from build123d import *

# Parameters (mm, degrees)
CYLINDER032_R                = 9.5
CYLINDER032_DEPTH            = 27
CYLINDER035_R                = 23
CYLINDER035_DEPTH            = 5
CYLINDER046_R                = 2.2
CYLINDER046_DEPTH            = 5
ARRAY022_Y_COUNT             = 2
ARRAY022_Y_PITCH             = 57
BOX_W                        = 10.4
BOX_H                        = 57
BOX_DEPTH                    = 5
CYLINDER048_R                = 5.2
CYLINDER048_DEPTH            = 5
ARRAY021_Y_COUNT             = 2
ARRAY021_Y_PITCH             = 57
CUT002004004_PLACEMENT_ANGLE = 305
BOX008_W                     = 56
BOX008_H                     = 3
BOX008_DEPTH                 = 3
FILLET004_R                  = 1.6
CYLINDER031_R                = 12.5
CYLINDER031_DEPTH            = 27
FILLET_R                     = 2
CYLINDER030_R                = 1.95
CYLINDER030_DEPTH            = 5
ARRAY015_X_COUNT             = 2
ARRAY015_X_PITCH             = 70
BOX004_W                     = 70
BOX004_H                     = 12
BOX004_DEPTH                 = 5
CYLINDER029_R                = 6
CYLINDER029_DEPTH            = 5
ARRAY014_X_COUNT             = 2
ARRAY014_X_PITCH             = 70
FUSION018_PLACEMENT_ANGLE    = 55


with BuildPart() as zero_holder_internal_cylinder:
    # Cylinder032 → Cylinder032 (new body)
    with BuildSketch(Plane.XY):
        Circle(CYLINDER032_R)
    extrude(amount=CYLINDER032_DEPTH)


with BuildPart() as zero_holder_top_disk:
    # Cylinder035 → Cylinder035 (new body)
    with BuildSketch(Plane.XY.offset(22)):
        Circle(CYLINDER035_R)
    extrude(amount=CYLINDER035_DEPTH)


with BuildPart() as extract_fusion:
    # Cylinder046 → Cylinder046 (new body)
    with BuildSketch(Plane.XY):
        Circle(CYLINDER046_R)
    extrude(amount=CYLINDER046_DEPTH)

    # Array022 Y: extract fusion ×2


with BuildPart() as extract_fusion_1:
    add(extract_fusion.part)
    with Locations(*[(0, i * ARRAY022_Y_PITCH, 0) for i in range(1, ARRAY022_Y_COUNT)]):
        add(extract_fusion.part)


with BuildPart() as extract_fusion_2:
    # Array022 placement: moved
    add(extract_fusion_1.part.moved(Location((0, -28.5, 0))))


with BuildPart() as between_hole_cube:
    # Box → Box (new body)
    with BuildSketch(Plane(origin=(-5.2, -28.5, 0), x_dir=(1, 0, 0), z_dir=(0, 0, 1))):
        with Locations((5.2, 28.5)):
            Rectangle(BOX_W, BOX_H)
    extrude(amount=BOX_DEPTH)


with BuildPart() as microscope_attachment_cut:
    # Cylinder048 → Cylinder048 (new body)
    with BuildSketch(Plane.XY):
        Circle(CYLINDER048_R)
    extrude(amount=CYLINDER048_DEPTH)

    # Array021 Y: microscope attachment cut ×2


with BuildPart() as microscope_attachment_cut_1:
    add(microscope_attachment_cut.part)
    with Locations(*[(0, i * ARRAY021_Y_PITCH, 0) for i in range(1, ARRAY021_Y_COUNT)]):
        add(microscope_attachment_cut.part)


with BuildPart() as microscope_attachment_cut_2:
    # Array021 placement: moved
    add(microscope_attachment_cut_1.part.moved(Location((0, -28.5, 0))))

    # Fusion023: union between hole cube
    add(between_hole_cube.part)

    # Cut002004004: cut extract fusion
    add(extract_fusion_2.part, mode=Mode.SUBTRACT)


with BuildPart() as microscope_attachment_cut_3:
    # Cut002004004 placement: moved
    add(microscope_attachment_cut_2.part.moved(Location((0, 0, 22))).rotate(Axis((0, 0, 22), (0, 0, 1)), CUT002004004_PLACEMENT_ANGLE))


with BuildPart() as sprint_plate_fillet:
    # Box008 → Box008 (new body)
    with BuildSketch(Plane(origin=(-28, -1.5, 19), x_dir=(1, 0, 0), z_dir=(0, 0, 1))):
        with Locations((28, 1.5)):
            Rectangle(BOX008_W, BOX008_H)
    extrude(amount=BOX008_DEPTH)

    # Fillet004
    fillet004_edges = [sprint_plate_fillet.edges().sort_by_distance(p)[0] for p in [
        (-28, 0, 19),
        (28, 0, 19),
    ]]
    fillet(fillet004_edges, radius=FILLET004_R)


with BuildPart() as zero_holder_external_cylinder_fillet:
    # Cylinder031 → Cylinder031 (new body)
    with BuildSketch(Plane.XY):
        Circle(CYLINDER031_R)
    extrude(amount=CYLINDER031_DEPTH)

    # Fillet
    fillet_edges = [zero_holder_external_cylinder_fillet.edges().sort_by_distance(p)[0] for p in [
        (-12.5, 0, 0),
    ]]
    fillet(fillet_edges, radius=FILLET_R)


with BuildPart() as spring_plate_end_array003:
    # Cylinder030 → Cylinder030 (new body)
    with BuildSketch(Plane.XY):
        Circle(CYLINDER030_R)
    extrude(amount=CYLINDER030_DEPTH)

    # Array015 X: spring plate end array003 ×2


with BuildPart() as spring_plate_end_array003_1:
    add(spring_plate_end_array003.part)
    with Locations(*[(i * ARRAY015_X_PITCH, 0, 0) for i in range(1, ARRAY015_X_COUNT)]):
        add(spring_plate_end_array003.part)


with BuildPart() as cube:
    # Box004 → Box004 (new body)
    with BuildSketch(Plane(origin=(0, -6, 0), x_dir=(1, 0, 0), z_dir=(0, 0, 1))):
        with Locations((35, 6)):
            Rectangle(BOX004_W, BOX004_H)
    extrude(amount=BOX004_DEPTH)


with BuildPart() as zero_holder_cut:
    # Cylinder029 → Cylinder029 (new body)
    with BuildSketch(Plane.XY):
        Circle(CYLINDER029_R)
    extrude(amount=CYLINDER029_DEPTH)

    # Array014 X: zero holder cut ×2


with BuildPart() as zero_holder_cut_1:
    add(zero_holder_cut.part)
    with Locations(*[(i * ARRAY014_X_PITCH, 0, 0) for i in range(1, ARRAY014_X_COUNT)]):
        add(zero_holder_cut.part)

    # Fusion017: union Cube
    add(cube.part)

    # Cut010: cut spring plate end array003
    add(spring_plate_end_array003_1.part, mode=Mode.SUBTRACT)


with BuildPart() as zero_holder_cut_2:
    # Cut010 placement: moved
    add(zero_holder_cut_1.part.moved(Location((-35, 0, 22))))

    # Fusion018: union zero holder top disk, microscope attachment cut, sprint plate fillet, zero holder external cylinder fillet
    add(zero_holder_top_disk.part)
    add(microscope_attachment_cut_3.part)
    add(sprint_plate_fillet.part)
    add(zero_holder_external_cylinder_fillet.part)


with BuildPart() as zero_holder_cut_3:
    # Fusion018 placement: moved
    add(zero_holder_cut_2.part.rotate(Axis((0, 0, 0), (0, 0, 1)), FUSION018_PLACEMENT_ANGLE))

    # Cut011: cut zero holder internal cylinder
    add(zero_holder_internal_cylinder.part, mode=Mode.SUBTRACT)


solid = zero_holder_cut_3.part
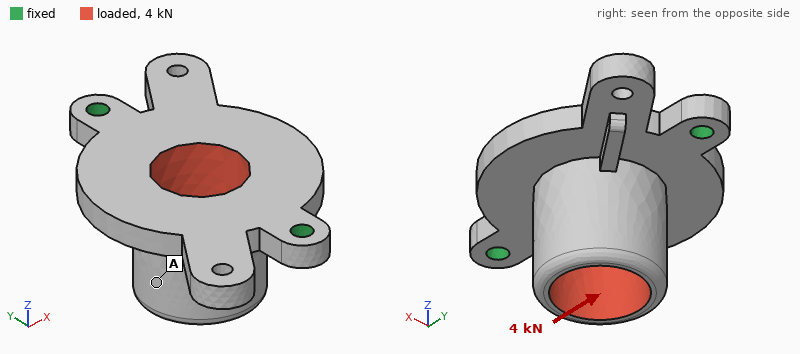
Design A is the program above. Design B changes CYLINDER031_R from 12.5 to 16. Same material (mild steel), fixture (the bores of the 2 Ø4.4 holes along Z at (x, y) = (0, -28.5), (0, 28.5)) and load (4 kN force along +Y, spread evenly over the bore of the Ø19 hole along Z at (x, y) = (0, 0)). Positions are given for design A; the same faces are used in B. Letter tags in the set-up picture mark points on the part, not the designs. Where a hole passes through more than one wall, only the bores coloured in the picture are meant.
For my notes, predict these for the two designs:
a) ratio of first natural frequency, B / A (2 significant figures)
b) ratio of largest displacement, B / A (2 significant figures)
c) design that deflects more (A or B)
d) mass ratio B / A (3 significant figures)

0.79
0.52
A
1.47
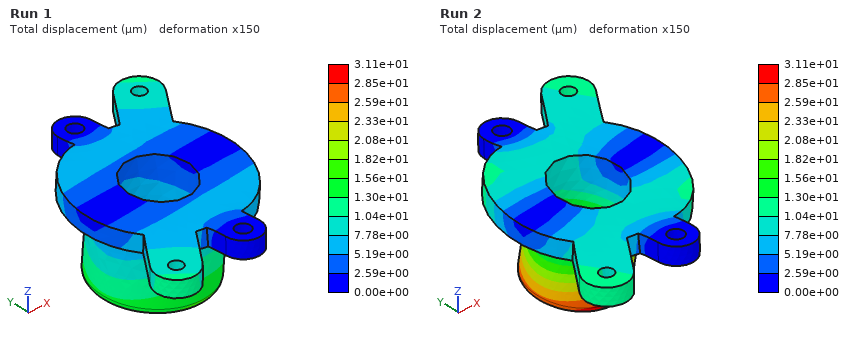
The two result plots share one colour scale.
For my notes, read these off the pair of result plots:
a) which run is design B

Run 1
